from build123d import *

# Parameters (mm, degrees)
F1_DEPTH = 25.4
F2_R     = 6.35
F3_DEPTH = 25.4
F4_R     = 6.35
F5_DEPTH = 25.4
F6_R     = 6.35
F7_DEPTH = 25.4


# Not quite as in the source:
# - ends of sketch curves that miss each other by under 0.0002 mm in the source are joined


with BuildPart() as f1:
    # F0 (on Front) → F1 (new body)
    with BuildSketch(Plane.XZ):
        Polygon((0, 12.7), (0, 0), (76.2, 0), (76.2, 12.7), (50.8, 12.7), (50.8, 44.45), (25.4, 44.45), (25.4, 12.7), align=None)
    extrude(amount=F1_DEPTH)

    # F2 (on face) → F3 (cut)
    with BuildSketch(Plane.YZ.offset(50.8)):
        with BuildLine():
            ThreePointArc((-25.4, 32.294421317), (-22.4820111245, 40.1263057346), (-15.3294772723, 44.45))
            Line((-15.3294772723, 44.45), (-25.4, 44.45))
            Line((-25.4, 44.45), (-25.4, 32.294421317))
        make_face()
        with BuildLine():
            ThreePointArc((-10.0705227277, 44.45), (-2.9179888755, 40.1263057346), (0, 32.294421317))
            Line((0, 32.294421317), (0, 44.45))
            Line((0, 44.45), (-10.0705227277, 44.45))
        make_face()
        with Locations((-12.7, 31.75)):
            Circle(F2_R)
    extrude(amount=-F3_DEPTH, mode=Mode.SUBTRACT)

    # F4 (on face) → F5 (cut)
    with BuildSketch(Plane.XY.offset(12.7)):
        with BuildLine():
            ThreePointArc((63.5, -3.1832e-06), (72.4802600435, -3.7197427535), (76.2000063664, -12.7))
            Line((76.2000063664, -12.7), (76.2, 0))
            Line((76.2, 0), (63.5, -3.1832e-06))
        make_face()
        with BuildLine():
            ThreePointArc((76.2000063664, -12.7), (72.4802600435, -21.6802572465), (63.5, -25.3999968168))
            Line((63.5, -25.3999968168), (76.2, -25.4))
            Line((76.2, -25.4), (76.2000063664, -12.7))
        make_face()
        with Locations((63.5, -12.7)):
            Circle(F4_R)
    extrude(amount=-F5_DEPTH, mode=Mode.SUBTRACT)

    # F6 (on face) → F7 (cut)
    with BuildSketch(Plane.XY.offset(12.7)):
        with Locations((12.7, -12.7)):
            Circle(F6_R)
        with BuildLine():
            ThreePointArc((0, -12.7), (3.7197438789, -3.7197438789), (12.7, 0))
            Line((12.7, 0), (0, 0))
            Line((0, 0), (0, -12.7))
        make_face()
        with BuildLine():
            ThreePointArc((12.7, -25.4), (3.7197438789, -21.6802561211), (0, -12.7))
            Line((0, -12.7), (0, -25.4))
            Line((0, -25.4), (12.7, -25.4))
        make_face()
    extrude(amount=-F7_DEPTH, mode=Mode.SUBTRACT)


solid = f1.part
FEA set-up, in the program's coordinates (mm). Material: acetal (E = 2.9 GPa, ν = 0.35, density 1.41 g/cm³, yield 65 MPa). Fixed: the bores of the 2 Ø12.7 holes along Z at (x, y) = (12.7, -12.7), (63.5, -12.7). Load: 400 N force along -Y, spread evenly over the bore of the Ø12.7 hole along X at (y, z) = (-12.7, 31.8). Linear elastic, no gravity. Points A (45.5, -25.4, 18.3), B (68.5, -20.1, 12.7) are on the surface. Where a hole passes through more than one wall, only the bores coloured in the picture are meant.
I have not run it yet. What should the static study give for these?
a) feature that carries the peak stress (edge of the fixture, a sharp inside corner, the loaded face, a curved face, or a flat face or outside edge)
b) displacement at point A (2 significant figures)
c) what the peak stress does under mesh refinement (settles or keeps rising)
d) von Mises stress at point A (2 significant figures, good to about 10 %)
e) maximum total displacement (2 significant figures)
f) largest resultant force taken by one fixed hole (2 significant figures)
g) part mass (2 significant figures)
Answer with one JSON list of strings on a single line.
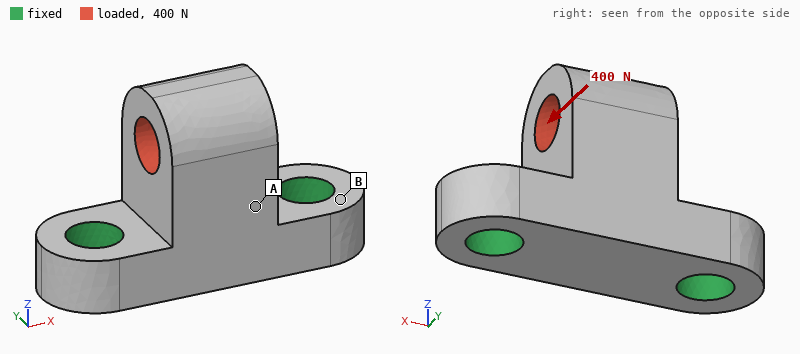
["edge of the fixture", "0.086 mm", "keeps rising", "2.4 MPa", "0.21 mm", "200 N", "50 g"]
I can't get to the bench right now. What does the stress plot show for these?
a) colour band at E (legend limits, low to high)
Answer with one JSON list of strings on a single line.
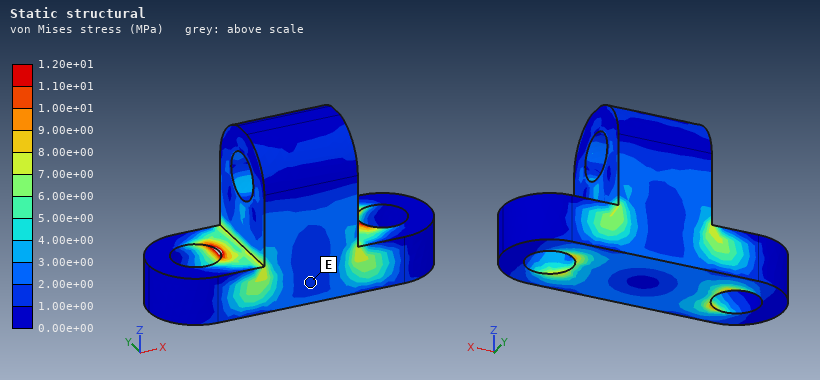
["1.00e+00 to 2.00e+00 MPa"]
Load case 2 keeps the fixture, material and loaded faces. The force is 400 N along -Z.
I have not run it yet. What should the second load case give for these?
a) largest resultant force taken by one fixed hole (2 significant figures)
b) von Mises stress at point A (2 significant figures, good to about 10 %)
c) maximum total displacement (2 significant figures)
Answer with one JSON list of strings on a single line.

["210 N", "0.84 MPa", "22 µm"]
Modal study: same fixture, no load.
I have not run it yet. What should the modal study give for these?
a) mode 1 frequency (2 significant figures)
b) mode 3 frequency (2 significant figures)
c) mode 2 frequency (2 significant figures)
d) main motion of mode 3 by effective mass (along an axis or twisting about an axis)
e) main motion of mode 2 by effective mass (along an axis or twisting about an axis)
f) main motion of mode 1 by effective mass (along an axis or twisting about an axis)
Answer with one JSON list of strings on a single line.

["1900 Hz", "4800 Hz", "3400 Hz", "along Z", "along X", "along Y"]
